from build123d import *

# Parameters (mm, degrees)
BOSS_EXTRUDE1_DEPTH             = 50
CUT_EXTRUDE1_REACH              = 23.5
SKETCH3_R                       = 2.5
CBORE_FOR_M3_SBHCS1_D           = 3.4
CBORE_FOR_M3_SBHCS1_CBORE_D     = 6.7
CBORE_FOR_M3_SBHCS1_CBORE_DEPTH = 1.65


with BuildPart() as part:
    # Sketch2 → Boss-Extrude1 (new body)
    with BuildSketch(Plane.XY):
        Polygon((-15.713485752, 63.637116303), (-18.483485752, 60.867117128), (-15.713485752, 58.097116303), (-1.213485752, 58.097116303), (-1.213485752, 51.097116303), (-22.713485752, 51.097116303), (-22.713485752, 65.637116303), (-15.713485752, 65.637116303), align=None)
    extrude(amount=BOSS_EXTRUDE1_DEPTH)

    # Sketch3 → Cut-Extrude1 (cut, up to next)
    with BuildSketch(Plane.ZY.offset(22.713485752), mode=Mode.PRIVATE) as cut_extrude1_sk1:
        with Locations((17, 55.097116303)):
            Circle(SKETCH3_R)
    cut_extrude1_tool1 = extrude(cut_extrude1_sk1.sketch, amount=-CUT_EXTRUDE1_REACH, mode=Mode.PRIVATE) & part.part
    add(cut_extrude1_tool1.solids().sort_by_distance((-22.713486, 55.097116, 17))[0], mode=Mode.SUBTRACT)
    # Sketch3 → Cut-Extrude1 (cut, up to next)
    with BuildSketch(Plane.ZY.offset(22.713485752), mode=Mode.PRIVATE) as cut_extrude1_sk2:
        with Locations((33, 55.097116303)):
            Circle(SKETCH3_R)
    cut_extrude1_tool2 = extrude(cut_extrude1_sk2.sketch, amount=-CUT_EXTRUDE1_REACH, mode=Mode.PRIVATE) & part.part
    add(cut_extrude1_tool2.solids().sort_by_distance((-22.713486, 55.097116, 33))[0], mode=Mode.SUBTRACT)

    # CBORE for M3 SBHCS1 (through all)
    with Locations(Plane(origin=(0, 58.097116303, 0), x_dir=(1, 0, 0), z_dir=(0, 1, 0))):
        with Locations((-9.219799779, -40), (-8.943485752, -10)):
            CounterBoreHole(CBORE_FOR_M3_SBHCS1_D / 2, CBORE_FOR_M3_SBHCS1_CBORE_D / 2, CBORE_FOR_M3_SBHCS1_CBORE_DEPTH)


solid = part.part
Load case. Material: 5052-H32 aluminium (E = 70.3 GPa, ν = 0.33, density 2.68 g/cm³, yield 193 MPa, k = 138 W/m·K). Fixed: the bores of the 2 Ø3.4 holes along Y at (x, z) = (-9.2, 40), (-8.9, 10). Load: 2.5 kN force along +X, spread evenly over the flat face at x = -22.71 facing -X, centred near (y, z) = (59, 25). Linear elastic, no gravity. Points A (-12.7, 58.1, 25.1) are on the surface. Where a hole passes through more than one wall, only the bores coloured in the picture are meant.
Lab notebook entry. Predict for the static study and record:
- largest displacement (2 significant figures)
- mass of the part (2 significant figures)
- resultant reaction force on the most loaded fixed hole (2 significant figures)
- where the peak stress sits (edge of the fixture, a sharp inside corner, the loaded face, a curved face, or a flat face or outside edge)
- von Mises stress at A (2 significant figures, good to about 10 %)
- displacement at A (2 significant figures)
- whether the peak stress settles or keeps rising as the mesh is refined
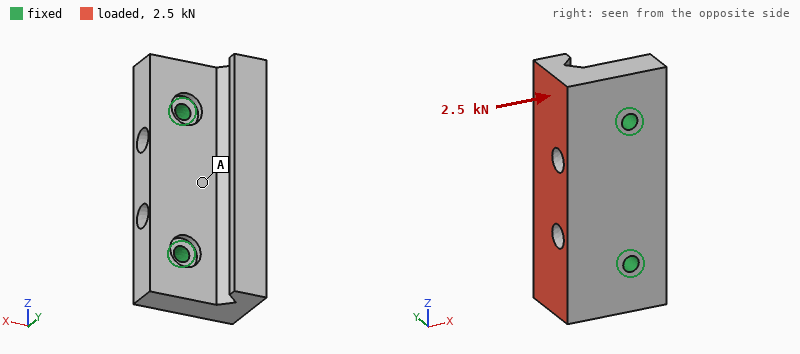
39 µm
23 g
1.3 kN
edge of the fixture
17 MPa
11 µm
keeps rising
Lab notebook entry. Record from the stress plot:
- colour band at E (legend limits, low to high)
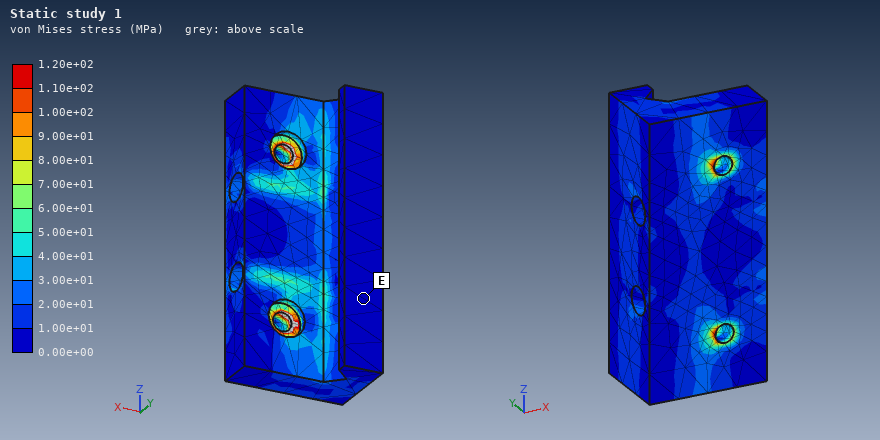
0.00e+00 to 1.00e+01 MPa
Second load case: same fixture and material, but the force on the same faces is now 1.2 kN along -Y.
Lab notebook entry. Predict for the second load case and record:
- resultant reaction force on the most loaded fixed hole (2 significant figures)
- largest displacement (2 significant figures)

600 N
43 µm
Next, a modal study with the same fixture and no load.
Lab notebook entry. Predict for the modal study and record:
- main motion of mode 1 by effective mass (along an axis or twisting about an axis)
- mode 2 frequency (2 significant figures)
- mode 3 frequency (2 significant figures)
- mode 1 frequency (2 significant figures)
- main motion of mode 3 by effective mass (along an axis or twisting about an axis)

along Y
14 kHz
21 kHz
9900 Hz
along Y
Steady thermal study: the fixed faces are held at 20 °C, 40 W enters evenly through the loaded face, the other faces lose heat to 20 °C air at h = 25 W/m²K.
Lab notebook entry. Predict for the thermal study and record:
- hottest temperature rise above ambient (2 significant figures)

19 K
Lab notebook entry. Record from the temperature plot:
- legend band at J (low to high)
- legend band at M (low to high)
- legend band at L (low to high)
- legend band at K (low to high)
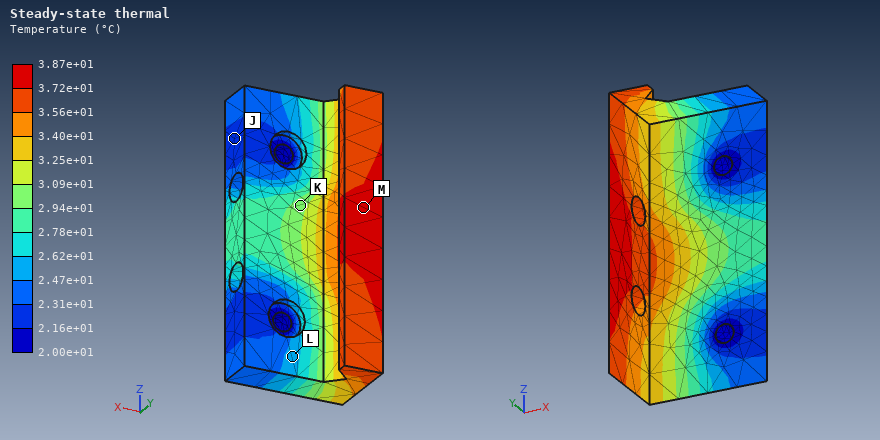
2.16e+01 to 2.31e+01 °C
3.72e+01 to 3.87e+01 °C
2.47e+01 to 2.62e+01 °C
2.94e+01 to 3.09e+01 °C
